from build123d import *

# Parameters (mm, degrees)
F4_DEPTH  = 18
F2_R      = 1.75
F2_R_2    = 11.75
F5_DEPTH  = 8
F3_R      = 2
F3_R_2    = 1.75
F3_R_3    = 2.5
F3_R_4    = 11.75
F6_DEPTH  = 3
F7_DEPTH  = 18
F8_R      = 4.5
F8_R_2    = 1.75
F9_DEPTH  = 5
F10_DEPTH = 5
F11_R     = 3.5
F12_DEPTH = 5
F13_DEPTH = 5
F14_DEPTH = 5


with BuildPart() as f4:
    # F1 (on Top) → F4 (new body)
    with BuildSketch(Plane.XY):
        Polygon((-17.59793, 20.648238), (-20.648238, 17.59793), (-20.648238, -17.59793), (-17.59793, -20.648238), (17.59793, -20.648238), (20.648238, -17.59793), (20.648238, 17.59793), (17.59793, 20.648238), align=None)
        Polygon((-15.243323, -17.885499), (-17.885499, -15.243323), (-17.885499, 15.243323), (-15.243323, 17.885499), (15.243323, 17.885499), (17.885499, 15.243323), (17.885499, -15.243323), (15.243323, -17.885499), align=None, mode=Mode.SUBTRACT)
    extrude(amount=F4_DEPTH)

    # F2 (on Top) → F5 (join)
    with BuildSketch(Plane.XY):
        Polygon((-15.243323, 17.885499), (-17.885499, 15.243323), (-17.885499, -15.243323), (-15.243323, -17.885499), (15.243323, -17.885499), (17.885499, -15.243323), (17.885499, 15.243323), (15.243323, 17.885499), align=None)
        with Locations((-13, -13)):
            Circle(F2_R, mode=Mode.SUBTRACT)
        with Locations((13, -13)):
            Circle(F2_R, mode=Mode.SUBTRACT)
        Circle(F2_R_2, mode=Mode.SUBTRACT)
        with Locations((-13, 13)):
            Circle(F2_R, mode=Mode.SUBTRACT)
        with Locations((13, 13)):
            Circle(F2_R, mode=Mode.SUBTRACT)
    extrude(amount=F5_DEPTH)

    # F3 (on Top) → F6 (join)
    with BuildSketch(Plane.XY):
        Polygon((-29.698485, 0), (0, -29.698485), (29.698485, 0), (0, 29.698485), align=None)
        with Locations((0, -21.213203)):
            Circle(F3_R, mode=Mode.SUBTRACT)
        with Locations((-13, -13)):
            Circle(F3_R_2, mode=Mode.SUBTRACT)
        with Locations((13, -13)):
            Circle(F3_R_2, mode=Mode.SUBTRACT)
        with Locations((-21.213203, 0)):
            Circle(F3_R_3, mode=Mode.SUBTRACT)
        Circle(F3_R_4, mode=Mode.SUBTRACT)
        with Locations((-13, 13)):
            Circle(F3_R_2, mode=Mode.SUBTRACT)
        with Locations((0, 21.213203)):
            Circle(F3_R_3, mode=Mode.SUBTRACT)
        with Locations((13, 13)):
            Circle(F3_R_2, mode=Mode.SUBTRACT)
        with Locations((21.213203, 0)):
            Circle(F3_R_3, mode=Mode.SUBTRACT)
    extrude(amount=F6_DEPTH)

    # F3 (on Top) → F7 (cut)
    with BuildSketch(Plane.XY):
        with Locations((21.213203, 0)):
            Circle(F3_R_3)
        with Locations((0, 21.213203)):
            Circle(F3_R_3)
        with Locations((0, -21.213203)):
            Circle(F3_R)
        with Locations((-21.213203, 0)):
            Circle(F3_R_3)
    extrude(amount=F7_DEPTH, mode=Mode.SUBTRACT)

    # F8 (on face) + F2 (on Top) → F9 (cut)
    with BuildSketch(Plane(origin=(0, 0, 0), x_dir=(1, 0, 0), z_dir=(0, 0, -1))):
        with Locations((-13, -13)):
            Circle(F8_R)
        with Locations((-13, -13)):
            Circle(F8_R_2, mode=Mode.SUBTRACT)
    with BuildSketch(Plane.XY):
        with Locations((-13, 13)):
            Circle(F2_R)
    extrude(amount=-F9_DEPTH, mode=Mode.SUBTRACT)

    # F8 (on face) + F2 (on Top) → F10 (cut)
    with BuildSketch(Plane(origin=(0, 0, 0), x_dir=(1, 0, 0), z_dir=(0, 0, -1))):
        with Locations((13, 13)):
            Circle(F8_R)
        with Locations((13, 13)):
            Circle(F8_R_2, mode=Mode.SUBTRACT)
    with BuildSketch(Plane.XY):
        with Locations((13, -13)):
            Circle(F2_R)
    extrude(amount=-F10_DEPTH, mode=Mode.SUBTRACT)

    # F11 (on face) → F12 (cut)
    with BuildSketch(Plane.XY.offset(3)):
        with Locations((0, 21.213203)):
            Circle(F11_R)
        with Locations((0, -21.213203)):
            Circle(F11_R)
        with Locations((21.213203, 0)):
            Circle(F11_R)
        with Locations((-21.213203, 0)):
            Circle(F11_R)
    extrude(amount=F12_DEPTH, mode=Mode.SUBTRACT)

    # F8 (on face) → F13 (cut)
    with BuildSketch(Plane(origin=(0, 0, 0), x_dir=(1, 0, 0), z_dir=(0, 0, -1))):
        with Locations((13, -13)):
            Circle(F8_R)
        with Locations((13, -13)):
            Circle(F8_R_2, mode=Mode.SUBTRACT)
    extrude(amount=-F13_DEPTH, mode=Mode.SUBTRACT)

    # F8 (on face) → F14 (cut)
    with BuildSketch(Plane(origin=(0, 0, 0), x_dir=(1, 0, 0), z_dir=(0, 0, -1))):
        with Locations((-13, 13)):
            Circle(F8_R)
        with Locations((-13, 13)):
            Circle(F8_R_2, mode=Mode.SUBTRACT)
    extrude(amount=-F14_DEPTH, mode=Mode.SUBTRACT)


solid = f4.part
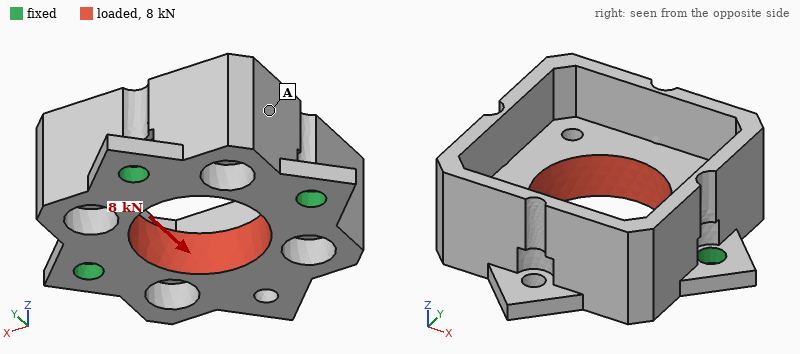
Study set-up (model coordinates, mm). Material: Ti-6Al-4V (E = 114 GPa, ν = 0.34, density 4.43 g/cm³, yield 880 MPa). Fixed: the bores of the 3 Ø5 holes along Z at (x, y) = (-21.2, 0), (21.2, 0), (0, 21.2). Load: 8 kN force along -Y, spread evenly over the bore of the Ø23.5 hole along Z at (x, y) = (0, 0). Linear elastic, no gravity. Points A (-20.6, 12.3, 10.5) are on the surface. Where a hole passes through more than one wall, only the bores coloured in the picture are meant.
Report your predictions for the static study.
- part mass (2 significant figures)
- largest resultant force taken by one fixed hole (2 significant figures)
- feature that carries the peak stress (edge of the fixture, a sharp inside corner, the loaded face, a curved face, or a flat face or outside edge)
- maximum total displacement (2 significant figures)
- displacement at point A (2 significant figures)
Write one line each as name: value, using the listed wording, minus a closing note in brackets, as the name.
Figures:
part mass: 58 g
largest resultant force taken by one fixed hole: 2.9 kN
feature that carries the peak stress: edge of the fixture
maximum total displacement: 26 µm
displacement at point A: 11 µm
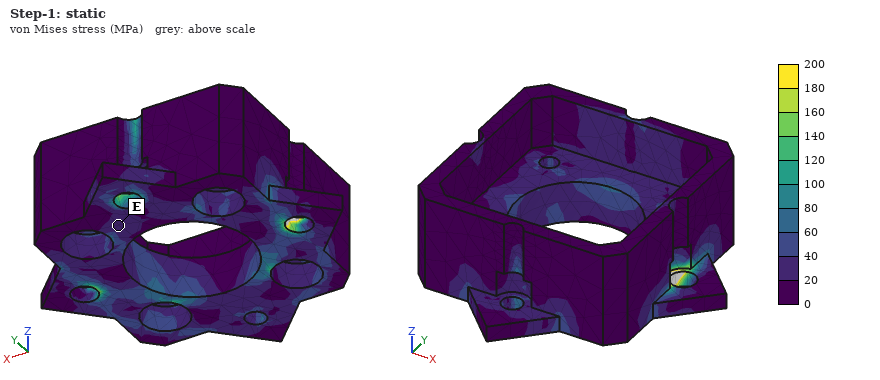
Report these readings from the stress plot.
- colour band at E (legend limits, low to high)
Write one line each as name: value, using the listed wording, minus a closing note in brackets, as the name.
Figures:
colour band at E: 20 to 40 MPa
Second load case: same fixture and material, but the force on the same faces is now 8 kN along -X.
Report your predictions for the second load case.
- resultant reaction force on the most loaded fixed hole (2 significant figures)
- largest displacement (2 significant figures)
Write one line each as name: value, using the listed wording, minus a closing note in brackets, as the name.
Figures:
resultant reaction force on the most loaded fixed hole: 3.3 kN
largest displacement: 17 µm
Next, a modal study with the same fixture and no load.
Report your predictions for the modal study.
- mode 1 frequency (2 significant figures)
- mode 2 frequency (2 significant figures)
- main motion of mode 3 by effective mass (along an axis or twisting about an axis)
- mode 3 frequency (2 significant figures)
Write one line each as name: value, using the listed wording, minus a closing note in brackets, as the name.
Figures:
mode 1 frequency: 6600 Hz
mode 2 frequency: 9800 Hz
main motion of mode 3 by effective mass: along X
mode 3 frequency: 15 kHz
